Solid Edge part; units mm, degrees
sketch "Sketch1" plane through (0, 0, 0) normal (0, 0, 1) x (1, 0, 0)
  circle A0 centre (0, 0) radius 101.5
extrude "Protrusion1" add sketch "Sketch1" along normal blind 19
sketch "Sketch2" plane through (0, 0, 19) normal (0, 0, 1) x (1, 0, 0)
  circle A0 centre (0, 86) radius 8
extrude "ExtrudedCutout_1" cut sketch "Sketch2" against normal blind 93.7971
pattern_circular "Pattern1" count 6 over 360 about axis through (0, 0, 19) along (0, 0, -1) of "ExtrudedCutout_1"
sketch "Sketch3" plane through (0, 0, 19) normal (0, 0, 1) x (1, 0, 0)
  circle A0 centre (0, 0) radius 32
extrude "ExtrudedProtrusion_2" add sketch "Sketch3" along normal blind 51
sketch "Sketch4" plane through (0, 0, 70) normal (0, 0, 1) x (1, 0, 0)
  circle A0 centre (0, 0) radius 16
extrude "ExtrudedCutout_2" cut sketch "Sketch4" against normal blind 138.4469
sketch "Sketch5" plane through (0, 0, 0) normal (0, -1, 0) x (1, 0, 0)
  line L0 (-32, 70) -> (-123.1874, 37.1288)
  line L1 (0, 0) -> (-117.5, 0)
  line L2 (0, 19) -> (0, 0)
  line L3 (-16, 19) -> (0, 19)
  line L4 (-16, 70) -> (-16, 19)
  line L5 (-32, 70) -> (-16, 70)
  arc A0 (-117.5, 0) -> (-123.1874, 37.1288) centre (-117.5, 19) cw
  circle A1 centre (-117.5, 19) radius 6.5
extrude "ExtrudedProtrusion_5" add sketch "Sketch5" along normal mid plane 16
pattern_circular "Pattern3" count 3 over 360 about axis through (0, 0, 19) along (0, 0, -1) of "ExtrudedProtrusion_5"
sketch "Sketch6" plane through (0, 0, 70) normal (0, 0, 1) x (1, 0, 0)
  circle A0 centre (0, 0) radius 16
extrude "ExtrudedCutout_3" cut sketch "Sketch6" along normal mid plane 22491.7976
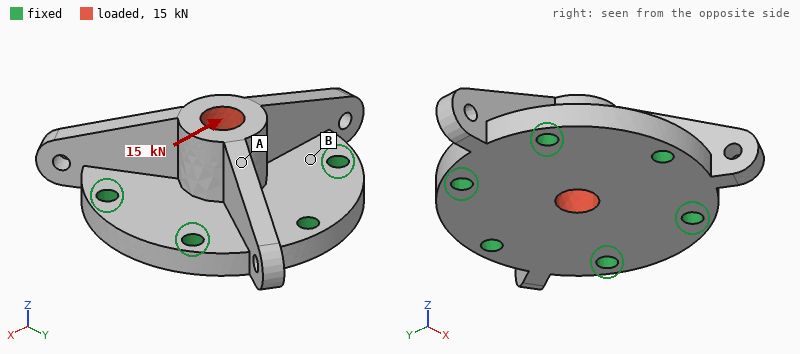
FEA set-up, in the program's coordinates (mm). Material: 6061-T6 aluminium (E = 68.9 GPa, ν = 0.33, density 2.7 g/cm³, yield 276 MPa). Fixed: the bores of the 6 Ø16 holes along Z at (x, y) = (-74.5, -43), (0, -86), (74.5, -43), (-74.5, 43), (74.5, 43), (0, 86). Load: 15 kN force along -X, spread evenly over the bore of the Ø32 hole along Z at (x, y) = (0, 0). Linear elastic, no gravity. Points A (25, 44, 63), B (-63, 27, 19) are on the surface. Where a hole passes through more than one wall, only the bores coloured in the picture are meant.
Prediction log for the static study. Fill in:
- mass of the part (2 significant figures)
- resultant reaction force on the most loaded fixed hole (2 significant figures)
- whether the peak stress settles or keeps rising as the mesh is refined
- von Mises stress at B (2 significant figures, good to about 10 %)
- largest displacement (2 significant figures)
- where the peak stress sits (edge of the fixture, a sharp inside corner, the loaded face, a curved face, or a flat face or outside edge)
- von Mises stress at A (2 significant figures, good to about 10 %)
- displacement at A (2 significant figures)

2.4 kg
3.9 kN
keeps rising
5.8 MPa
19 µm
edge of the fixture
2.2 MPa
10 µm
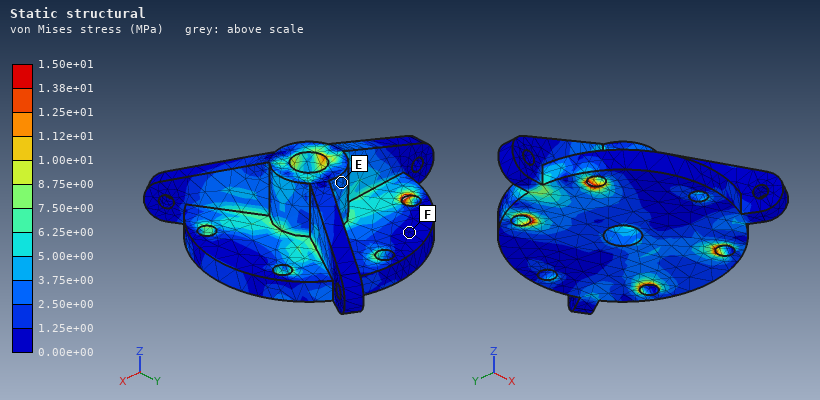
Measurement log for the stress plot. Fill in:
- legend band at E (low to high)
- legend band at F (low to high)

2.50e+00 to 3.75e+00 MPa
0.00e+00 to 1.25e+00 MPa
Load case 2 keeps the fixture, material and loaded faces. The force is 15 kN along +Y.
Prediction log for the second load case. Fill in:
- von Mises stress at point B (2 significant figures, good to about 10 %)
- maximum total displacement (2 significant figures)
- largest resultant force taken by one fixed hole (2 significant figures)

3.5 MPa
17 µm
4.2 kN
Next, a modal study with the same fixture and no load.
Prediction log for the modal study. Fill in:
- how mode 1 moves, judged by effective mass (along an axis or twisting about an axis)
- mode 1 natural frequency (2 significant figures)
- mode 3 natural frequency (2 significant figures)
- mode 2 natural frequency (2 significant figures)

along Z
5100 Hz
5400 Hz
5400 Hz
